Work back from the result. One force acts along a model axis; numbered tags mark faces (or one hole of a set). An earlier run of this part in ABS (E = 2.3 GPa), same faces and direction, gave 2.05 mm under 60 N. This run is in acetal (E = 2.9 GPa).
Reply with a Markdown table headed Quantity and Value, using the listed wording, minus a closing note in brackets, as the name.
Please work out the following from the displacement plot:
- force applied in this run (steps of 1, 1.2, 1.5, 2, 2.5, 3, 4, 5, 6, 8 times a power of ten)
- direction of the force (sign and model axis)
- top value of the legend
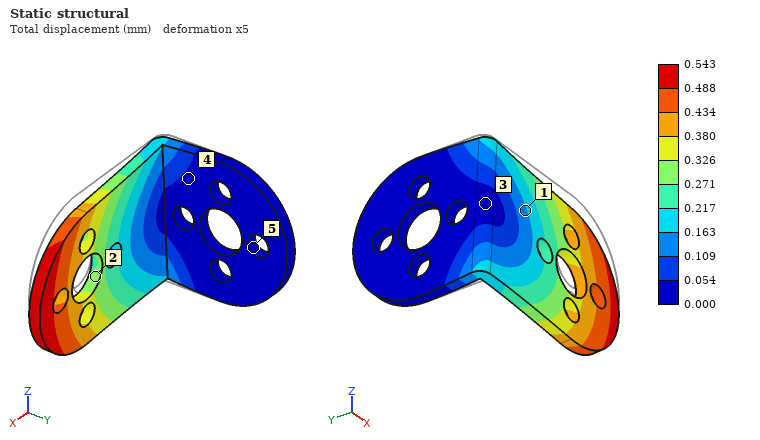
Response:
| Quantity | Value |
|---|---|
| force applied in this run | 20 N |
| direction of the force | -Z |
| top value of the legend | 0.543 mm |
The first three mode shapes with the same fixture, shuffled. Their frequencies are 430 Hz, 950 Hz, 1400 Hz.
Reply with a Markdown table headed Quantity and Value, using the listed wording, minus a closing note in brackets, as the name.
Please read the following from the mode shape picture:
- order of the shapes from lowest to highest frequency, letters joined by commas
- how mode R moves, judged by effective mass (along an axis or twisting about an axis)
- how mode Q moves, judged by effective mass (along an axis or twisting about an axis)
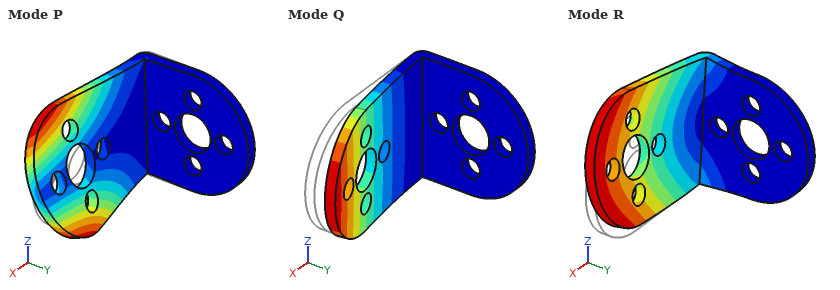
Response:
| Quantity | Value |
|---|---|
| order of the shapes from lowest to highest frequency, letters joined by commas | Q, R, P |
| how mode R moves, judged by effective mass | along Z |
| how mode Q moves, judged by effective mass | along Y |
